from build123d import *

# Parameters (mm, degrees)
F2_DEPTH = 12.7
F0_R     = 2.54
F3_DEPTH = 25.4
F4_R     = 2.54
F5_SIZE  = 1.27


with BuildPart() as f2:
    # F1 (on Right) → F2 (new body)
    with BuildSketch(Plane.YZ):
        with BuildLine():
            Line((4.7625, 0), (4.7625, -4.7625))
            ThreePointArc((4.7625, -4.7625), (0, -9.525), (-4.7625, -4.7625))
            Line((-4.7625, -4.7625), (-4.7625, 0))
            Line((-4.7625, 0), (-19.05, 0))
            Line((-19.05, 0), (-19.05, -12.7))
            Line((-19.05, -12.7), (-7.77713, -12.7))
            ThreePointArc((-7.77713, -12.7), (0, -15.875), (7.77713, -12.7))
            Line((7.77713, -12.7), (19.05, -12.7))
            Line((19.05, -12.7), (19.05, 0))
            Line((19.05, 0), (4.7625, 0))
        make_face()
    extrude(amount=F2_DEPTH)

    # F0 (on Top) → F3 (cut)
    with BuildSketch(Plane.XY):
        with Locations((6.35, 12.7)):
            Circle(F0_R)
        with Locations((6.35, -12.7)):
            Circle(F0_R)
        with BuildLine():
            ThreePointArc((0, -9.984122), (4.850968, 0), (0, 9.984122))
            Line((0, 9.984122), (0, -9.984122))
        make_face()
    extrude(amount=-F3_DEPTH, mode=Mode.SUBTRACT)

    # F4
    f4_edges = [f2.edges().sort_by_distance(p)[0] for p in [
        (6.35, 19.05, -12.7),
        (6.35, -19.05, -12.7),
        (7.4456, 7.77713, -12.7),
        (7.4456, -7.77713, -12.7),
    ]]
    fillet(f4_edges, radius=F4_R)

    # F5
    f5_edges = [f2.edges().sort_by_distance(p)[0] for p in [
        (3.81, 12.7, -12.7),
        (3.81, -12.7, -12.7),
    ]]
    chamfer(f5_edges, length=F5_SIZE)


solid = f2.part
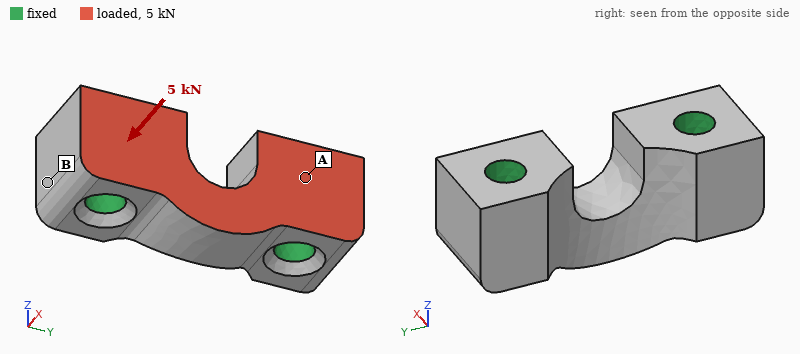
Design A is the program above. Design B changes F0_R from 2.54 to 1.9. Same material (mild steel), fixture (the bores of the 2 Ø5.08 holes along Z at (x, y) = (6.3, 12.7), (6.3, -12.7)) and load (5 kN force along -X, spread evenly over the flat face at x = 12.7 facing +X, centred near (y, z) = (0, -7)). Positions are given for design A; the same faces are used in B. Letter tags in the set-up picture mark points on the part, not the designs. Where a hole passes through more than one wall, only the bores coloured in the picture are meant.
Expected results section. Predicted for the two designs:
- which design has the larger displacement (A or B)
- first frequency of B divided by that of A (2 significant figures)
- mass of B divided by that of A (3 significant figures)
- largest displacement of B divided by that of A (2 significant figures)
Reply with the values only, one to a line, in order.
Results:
B
0.85
1.05
1.2
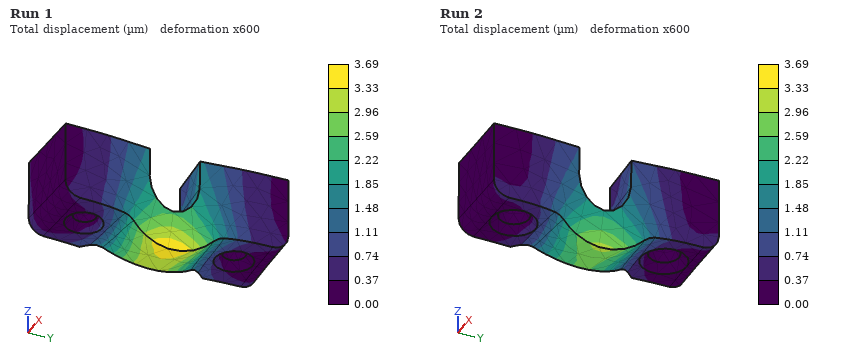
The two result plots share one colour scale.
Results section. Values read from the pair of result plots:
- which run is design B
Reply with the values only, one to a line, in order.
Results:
Run 1
